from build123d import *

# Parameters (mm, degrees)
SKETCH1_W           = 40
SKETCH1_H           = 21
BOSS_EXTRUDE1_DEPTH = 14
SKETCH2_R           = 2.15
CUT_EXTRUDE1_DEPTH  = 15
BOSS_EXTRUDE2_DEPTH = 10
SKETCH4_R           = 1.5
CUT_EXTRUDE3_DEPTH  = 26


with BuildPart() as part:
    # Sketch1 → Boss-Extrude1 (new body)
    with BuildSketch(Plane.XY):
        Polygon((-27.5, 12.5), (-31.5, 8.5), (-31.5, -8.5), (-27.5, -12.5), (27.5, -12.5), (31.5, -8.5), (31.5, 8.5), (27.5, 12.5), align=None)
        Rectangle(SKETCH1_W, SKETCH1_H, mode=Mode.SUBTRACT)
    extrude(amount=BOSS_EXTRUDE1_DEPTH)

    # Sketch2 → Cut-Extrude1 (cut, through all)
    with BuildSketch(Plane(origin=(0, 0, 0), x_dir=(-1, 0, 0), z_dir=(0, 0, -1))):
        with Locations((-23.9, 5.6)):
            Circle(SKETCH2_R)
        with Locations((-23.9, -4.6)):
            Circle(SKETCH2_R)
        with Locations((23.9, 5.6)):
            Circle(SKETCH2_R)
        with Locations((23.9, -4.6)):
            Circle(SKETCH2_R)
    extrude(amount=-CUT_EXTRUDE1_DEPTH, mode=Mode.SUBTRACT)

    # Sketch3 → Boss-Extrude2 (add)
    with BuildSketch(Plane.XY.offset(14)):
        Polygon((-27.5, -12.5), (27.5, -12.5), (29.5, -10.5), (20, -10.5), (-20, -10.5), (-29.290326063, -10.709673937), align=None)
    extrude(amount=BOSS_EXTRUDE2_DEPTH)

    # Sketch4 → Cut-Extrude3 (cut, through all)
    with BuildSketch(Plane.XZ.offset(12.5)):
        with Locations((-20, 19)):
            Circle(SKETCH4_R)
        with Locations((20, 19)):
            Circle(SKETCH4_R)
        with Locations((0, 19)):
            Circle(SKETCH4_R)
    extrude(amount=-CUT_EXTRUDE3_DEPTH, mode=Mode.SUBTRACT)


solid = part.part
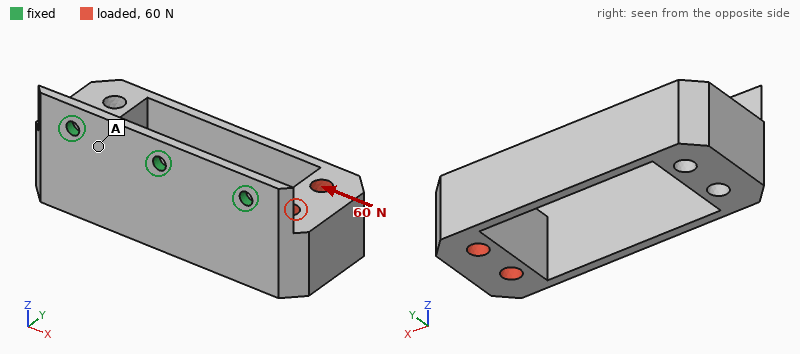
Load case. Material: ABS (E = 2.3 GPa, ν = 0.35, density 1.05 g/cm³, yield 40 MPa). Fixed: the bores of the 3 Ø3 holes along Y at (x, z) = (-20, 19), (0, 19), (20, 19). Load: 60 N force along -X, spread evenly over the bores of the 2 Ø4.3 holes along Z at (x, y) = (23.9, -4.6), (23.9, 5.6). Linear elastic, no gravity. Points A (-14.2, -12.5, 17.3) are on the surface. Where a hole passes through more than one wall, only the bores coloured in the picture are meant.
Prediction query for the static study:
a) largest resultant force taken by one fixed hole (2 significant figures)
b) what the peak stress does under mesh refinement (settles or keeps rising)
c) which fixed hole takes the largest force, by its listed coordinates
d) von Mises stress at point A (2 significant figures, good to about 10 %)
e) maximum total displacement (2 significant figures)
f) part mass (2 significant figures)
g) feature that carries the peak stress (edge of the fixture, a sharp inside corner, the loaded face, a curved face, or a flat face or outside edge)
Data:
32 N
keeps rising
(20, 19)
2.6 MPa
0.81 mm
11 g
edge of the fixture
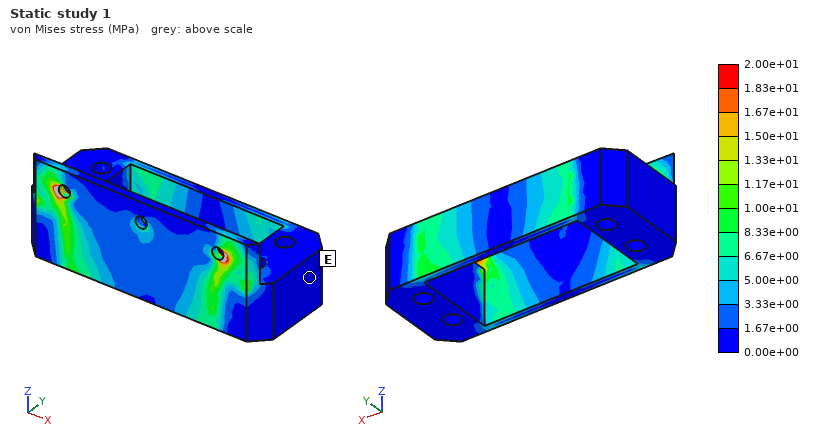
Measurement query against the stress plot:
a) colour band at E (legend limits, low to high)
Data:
0.00e+00 to 1.67e+00 MPa
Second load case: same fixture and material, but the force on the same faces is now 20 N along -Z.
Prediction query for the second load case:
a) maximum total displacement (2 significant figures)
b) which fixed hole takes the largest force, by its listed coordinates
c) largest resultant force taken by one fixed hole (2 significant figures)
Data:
0.76 mm
(20, 19)
22 N
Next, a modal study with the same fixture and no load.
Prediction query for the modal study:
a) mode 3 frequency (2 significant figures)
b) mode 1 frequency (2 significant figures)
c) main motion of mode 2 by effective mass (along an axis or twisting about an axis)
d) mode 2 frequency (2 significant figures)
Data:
990 Hz
310 Hz
along X
500 Hz
